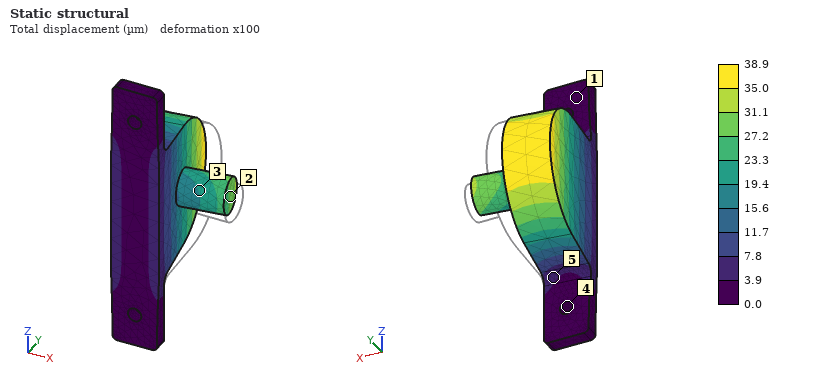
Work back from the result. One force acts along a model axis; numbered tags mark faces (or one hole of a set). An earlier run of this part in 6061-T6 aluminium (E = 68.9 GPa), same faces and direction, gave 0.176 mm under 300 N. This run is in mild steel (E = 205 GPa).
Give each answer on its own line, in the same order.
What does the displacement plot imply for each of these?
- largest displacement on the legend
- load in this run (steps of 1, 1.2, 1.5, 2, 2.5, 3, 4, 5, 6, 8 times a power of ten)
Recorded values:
38.9 µm
200 N
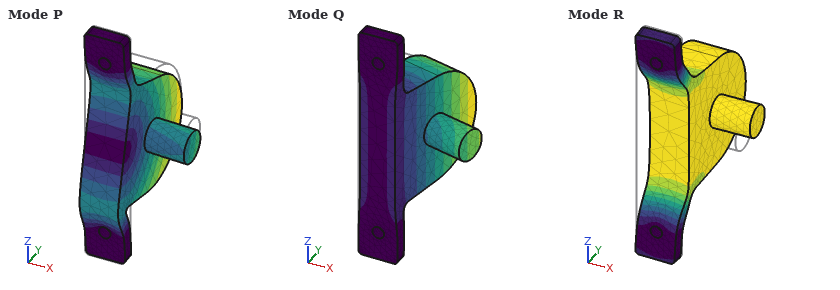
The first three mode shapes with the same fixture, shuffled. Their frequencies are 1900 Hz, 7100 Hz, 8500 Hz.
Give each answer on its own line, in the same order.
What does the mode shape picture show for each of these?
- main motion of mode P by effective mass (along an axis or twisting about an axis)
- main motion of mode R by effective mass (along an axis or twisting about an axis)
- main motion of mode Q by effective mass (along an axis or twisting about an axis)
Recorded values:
along Z
along Y
along X
